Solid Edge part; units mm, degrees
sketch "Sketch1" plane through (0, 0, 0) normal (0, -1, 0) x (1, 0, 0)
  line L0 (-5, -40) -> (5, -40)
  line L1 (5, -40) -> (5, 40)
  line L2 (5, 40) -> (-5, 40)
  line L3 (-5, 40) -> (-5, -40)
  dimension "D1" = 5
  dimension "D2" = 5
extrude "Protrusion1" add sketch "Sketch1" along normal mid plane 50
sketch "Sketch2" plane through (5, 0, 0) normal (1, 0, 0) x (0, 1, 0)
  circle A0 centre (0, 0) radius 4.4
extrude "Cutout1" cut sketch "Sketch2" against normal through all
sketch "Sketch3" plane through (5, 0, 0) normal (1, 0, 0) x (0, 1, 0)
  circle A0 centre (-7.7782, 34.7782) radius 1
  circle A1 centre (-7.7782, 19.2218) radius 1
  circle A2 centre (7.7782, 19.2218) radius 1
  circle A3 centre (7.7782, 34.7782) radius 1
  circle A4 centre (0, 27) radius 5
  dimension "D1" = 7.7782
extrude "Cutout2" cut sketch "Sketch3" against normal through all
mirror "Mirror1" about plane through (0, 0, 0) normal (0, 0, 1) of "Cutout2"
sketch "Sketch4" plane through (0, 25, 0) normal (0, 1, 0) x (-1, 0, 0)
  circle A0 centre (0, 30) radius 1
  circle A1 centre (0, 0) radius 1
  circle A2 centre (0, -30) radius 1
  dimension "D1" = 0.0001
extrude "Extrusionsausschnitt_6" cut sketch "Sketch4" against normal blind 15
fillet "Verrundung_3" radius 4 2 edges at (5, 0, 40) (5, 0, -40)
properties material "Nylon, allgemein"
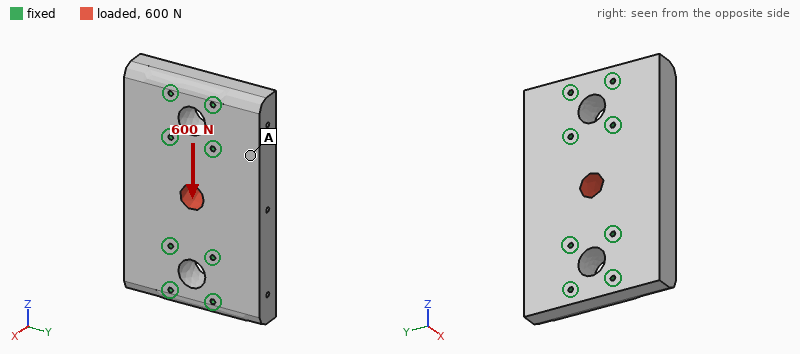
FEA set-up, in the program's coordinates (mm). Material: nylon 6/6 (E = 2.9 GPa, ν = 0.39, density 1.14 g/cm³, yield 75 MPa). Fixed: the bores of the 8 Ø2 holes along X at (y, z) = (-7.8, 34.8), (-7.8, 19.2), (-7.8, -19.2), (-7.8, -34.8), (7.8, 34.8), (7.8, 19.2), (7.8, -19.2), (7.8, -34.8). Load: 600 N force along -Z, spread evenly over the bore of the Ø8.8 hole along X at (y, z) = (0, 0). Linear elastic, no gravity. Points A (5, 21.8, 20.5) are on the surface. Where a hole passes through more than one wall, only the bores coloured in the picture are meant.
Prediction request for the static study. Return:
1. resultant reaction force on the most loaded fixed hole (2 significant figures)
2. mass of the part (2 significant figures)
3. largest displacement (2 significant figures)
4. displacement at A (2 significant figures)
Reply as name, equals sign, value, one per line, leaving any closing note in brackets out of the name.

resultant reaction force on the most loaded fixed hole = 140 N
mass of the part = 42 g
largest displacement = 11 µm
displacement at A = 2.6 µm
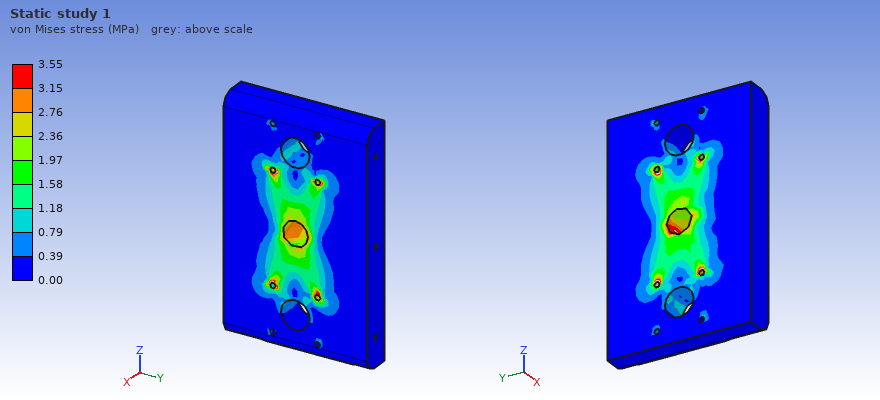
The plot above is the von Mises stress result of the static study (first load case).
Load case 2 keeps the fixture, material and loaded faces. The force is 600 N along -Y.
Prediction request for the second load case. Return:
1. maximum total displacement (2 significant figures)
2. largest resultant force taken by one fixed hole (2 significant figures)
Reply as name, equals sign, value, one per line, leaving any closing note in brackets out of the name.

maximum total displacement = 18 µm
largest resultant force taken by one fixed hole = 160 N
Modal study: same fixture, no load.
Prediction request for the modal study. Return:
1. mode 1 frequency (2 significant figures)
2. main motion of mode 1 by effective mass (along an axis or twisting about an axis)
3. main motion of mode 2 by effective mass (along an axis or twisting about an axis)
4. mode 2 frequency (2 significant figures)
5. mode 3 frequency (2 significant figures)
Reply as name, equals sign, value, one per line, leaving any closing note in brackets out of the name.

mode 1 frequency = 4600 Hz
main motion of mode 1 by effective mass = twisting about Z
main motion of mode 2 by effective mass = along X
mode 2 frequency = 4900 Hz
mode 3 frequency = 6500 Hz
